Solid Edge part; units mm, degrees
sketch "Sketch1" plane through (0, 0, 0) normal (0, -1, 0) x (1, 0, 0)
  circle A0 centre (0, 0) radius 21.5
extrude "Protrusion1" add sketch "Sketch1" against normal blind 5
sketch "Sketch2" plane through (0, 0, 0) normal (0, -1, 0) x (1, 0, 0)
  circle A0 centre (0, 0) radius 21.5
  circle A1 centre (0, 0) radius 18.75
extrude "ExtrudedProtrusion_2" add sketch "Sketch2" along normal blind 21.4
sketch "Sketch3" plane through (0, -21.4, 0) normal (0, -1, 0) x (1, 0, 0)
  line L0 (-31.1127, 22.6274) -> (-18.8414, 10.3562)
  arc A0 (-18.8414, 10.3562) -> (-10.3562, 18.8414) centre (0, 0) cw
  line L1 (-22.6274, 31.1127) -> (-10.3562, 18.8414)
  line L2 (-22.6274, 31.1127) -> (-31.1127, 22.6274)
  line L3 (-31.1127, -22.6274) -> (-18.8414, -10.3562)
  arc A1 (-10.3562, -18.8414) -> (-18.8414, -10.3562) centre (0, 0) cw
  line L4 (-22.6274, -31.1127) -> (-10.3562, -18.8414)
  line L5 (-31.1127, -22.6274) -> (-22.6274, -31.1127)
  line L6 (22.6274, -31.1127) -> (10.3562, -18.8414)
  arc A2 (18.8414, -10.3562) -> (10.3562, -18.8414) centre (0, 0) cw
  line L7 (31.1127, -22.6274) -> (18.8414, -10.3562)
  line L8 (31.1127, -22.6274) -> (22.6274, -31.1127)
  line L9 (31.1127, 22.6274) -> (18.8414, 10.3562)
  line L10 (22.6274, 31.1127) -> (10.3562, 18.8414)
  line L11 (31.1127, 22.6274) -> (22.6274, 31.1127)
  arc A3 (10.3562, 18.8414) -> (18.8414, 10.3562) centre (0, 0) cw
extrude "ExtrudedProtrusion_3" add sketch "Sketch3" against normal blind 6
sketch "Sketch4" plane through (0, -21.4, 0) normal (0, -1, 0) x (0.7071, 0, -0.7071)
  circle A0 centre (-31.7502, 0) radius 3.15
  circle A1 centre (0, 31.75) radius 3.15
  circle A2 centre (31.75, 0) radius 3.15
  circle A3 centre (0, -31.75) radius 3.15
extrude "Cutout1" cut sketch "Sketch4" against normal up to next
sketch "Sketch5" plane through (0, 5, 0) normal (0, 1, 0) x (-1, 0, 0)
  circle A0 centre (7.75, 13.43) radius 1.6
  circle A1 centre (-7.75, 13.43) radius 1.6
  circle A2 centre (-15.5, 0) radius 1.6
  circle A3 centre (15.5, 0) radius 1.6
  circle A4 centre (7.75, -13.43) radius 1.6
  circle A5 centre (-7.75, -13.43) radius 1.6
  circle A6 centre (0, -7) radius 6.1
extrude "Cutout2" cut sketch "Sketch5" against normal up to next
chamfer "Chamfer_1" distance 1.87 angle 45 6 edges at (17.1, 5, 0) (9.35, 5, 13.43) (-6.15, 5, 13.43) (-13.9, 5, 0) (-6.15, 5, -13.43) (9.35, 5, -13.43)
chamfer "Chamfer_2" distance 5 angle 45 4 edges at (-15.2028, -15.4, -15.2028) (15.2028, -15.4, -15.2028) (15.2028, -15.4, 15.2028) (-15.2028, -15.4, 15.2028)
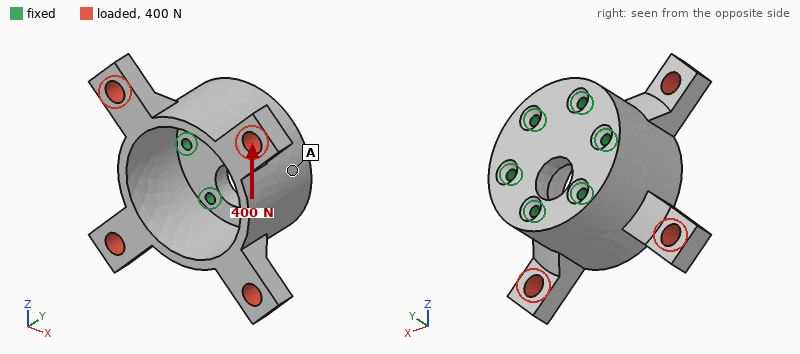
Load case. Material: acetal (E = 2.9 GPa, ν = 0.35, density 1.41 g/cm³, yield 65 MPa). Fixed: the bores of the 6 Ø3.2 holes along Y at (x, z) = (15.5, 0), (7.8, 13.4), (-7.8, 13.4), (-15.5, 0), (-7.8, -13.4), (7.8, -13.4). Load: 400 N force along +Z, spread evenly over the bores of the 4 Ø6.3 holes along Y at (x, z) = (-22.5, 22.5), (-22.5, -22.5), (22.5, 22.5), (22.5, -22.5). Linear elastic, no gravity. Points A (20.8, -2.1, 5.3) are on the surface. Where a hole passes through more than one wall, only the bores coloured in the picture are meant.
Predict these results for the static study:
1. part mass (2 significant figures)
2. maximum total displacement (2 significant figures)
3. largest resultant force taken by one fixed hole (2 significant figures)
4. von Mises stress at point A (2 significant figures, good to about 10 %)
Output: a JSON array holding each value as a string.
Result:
["26 g", "0.39 mm", "140 N", "2.3 MPa"]
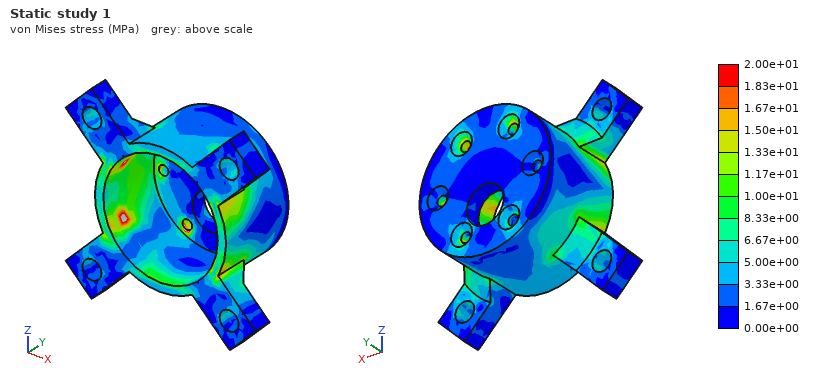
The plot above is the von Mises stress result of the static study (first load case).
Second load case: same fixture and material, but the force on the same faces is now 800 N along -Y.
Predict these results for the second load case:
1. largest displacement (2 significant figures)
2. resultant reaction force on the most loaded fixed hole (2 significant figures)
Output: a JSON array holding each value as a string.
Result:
["0.65 mm", "140 N"]
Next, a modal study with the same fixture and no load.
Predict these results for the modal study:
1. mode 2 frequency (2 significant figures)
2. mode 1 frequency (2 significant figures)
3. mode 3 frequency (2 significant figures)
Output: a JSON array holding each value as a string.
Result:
["2200 Hz", "1500 Hz", "2200 Hz"]
